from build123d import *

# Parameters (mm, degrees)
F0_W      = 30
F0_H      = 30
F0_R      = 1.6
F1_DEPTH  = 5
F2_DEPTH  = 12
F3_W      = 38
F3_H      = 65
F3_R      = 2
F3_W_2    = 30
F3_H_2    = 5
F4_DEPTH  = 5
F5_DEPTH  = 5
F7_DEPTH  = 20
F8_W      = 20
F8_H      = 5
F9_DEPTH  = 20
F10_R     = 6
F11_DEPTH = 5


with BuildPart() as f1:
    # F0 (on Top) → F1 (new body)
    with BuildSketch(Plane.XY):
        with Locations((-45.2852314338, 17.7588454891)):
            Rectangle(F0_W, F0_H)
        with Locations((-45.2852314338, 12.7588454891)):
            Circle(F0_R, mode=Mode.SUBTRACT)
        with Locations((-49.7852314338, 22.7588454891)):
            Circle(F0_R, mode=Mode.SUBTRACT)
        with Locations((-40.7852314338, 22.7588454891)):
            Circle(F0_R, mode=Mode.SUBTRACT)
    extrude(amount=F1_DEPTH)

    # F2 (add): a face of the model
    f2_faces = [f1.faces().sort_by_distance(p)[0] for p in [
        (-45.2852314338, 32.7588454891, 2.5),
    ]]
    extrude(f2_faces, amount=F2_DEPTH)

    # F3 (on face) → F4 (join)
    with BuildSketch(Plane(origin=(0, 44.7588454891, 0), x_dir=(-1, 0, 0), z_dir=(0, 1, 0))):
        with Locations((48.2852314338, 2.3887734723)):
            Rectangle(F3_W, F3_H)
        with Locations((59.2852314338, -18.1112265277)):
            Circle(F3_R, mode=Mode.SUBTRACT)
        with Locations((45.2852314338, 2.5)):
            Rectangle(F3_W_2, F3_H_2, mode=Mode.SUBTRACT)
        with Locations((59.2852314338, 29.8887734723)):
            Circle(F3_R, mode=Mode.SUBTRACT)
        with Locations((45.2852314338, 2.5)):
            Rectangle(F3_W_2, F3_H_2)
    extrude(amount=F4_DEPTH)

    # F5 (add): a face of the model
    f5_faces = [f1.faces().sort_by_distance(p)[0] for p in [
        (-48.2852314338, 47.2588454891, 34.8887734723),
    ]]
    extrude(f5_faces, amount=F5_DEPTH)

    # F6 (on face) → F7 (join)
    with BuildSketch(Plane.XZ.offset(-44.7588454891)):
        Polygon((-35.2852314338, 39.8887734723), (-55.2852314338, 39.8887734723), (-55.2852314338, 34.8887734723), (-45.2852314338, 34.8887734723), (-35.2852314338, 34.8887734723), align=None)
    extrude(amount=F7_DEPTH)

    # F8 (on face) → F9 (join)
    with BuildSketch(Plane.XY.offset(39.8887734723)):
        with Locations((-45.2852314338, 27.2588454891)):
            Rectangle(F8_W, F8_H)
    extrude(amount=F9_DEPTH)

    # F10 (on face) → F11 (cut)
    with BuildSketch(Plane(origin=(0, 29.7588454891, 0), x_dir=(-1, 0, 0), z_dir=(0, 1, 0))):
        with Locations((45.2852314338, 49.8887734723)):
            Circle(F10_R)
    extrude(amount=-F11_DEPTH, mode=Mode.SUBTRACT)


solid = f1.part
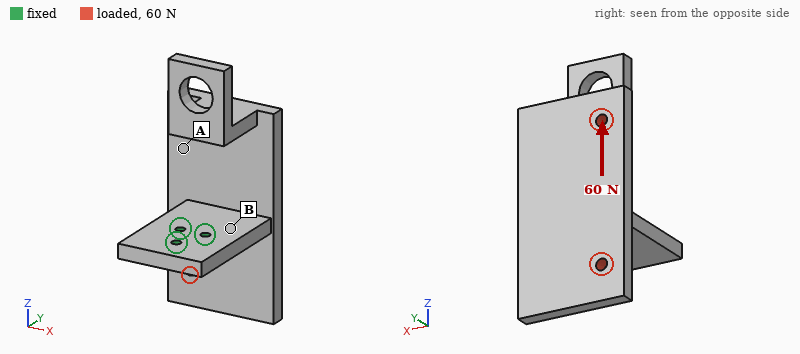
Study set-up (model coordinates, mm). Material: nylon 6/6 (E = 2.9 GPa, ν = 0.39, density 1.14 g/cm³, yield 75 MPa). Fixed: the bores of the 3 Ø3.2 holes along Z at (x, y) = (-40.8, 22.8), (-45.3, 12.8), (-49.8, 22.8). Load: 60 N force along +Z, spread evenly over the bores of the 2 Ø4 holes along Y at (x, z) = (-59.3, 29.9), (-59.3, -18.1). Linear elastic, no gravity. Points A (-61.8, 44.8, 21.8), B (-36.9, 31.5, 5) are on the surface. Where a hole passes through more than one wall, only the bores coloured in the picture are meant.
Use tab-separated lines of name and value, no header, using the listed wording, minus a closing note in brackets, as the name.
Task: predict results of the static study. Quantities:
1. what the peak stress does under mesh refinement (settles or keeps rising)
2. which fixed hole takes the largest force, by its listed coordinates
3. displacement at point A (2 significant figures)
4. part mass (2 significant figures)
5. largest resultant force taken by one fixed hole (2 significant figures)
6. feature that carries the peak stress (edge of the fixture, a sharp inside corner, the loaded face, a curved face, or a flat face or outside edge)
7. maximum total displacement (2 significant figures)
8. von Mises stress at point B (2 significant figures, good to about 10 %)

what the peak stress does under mesh refinement	keeps rising
which fixed hole takes the largest force, by its listed coordinates	(-49.8, 22.8)
displacement at point A	0.63 mm
part mass	26 g
largest resultant force taken by one fixed hole	98 N
feature that carries the peak stress	edge of the fixture
maximum total displacement	1.3 mm
von Mises stress at point B	7.2 MPa
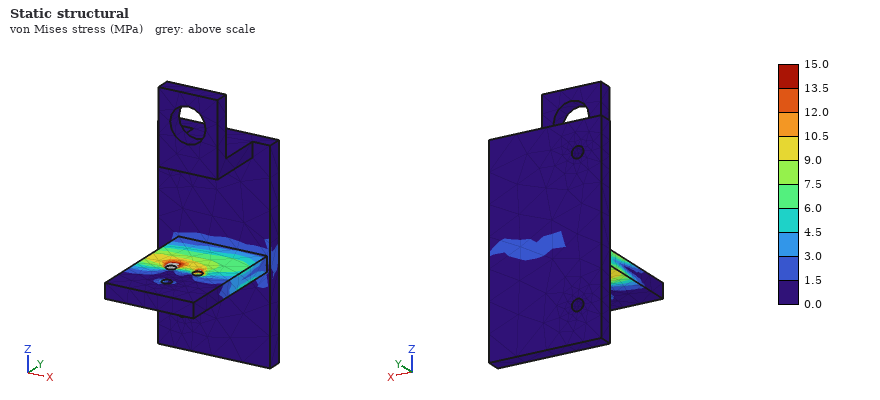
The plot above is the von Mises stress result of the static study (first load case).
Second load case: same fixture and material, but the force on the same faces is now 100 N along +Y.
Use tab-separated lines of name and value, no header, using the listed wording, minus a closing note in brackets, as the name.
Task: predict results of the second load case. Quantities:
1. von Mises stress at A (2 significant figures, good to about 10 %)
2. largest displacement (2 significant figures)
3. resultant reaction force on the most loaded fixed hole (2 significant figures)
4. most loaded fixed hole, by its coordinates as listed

von Mises stress at A	3.2 MPa
largest displacement	1.3 mm
resultant reaction force on the most loaded fixed hole	130 N
most loaded fixed hole, by its coordinates as listed	(-49.8, 22.8)
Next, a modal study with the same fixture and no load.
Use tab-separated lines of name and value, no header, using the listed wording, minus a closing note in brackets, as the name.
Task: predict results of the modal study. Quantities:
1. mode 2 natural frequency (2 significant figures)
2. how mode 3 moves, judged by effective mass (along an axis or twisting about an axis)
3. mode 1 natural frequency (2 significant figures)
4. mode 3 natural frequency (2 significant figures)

mode 2 natural frequency	350 Hz
how mode 3 moves, judged by effective mass	along Z
mode 1 natural frequency	240 Hz
mode 3 natural frequency	590 Hz
